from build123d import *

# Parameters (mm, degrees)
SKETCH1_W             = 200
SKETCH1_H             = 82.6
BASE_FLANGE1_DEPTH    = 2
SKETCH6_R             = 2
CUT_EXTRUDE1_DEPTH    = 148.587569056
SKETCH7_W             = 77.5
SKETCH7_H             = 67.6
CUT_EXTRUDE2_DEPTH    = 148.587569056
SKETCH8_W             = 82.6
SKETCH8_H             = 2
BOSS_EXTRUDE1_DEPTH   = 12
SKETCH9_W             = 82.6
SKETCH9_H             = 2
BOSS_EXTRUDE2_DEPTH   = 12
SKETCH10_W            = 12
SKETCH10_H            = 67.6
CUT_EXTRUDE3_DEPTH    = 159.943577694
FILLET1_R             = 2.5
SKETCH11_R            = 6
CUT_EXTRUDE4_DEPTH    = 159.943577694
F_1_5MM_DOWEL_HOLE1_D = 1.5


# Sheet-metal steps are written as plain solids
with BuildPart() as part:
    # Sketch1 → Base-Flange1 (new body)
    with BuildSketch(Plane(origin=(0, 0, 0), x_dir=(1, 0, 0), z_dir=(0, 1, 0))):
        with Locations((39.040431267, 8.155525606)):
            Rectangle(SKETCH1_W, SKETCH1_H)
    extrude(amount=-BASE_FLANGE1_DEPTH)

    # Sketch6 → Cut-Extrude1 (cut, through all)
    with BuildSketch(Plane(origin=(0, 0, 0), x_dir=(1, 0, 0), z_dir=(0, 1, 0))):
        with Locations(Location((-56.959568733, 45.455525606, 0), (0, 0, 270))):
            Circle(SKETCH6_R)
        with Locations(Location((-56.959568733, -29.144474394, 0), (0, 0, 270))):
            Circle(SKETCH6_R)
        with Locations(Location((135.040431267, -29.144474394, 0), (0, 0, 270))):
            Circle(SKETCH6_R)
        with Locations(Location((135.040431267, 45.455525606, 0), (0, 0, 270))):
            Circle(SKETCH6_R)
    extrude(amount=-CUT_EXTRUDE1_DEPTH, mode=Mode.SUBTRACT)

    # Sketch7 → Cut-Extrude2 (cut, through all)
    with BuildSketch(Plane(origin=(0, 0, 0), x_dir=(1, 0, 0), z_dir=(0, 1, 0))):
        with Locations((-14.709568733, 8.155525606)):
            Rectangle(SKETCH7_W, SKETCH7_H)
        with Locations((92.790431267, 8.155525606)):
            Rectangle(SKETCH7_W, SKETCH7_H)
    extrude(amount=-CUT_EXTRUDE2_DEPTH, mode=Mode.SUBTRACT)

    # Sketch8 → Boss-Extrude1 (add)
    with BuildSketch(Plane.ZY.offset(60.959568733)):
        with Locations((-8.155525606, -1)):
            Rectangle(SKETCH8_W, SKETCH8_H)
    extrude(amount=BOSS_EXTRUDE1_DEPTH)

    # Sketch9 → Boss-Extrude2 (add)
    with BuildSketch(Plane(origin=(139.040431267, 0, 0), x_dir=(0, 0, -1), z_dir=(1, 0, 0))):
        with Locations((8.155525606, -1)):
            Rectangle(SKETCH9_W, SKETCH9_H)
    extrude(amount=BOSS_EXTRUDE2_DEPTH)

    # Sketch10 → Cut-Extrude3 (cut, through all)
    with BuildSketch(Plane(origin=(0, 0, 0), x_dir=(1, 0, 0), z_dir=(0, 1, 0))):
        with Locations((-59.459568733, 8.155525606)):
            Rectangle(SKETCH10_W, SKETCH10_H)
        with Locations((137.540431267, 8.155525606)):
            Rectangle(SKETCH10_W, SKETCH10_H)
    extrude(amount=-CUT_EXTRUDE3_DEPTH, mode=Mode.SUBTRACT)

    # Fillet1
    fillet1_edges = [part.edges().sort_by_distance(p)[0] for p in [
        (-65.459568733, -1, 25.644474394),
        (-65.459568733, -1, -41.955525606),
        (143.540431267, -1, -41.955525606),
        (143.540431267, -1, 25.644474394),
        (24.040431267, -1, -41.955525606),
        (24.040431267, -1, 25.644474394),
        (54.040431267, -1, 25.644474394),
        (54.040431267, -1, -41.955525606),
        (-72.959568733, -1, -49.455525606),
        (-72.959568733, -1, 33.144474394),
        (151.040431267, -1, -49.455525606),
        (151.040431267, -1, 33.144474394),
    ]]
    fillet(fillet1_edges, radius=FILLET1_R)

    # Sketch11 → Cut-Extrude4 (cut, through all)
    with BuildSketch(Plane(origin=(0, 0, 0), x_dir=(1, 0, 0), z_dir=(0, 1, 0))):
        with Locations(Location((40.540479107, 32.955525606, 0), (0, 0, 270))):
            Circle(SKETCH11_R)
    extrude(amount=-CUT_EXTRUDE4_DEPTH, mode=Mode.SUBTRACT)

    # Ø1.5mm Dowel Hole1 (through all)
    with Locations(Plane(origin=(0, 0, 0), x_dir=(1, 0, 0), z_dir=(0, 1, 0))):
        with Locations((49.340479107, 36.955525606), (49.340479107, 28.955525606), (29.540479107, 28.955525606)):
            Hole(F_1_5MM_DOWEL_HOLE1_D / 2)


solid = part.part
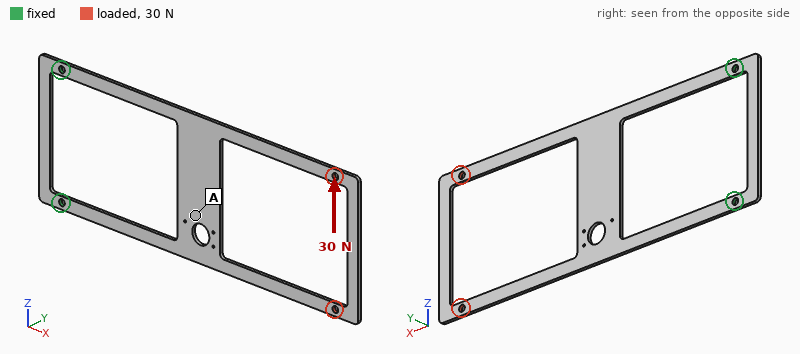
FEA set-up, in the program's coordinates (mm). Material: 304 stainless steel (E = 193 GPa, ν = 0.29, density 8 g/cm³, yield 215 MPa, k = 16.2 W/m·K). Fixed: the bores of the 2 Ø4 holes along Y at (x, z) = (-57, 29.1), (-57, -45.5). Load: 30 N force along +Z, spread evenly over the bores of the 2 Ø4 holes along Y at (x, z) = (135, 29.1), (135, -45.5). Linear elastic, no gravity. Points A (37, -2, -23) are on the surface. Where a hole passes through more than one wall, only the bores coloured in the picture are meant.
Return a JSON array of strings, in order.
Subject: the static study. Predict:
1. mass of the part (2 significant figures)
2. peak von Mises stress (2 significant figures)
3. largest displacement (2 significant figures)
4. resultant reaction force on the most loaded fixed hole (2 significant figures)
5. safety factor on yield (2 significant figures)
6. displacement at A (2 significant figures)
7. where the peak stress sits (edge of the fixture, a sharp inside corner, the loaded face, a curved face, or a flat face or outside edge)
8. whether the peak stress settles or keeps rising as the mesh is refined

["100 g", "55 MPa", "0.17 mm", "62 N", "3.9", "0.059 mm", "a curved face", "settles"]
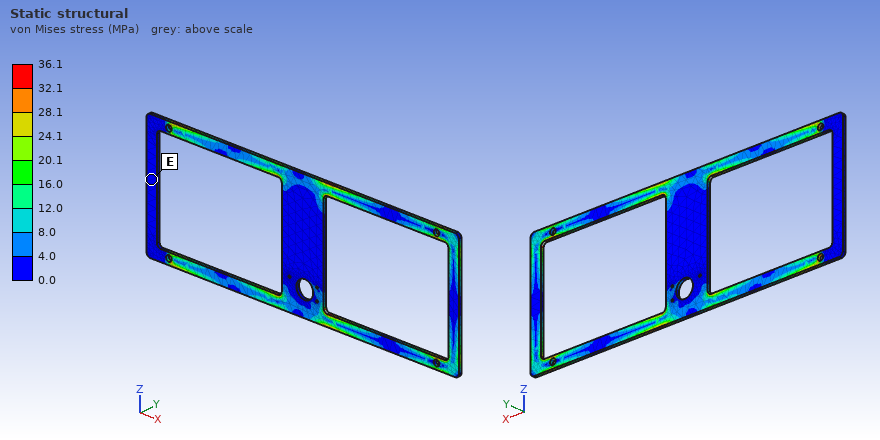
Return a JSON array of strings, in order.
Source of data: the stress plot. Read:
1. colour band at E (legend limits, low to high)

["0.0 to 4.0 MPa"]
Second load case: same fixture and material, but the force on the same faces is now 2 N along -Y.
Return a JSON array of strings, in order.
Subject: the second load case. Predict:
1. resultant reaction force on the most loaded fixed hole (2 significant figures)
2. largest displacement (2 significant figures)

["1.0 N", "2.5 mm"]
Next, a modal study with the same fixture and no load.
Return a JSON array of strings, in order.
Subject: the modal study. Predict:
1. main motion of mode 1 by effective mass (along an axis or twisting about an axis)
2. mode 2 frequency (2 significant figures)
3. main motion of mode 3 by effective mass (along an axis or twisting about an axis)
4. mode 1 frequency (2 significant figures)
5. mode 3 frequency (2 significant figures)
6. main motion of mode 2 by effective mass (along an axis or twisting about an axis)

["along Y", "140 Hz", "along Y", "28 Hz", "150 Hz", "twisting about X"]
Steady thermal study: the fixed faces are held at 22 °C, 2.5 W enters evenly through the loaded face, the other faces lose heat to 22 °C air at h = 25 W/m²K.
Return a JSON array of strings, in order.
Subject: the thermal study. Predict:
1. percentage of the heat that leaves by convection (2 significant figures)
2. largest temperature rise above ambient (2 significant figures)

["100 %", "58 K"]
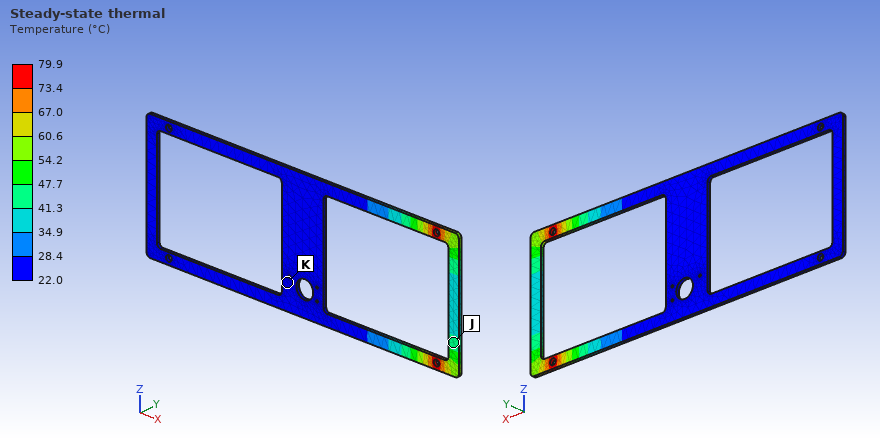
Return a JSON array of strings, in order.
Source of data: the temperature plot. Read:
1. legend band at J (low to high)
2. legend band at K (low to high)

["41.3 to 47.7 °C", "22.0 to 28.4 °C"]
